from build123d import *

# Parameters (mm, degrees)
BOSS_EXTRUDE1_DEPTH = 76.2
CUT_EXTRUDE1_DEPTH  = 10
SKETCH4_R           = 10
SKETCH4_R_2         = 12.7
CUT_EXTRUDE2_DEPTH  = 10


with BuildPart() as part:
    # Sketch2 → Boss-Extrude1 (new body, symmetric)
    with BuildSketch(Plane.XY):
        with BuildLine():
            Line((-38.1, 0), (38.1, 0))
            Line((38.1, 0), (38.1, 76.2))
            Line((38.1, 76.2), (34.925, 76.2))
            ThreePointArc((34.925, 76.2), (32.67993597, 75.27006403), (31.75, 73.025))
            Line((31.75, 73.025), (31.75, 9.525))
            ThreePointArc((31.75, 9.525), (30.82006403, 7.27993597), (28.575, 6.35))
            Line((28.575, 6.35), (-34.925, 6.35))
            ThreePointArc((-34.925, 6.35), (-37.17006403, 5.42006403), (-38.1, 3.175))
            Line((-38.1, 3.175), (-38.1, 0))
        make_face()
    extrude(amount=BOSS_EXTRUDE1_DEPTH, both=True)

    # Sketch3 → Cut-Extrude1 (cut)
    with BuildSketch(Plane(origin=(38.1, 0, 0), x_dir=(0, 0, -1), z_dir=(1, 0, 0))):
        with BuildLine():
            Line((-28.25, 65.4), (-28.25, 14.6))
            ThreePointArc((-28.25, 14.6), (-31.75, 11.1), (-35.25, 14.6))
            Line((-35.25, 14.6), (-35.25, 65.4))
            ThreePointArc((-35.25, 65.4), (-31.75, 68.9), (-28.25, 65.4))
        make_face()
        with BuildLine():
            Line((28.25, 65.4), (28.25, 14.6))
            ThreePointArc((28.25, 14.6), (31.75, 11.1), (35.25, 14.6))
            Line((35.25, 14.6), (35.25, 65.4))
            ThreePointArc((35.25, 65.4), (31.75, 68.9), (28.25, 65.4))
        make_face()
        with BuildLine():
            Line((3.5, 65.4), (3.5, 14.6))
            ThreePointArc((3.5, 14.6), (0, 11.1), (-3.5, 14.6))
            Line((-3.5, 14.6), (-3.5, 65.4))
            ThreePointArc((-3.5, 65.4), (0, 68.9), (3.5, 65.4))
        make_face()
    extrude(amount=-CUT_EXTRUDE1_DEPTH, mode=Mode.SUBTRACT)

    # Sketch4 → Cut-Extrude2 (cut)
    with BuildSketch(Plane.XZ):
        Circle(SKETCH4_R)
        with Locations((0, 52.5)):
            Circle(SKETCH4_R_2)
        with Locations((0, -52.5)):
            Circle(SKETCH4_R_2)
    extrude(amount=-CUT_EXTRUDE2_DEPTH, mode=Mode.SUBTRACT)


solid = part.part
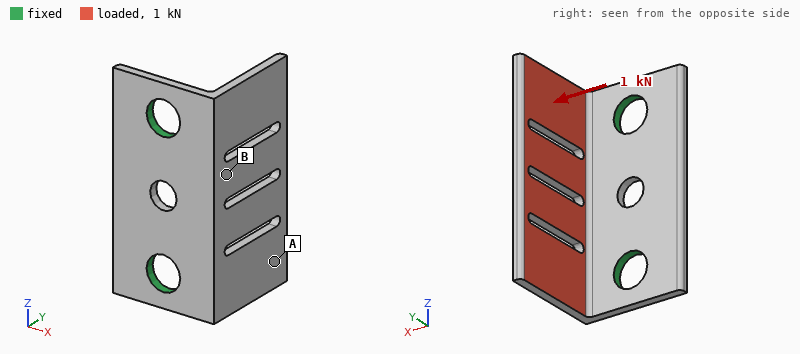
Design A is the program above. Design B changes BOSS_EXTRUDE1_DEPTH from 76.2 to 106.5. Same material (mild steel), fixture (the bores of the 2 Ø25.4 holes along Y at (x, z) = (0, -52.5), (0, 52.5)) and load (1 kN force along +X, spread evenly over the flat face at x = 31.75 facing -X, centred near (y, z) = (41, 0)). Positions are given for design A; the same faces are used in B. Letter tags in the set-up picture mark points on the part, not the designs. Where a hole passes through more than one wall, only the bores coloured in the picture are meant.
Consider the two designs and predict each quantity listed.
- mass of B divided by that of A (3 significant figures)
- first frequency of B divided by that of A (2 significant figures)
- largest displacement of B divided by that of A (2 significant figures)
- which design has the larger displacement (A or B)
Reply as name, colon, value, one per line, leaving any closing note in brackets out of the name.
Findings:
mass of B divided by that of A: 1.45
first frequency of B divided by that of A: 0.97
largest displacement of B divided by that of A: 0.73
which design has the larger displacement: A
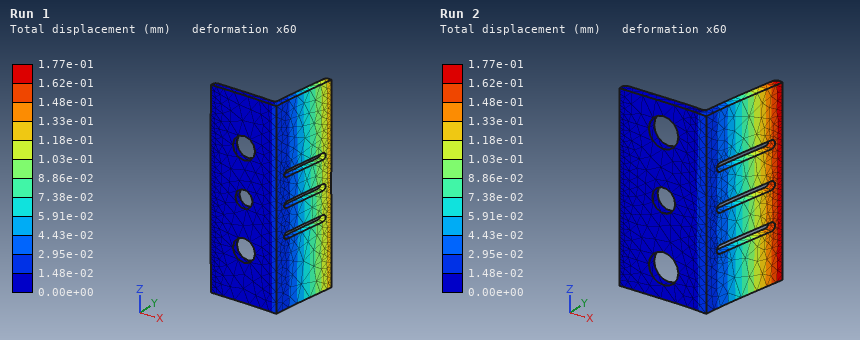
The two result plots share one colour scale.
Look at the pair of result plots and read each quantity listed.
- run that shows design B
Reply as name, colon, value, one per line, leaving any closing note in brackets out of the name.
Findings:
run that shows design B: Run 1
